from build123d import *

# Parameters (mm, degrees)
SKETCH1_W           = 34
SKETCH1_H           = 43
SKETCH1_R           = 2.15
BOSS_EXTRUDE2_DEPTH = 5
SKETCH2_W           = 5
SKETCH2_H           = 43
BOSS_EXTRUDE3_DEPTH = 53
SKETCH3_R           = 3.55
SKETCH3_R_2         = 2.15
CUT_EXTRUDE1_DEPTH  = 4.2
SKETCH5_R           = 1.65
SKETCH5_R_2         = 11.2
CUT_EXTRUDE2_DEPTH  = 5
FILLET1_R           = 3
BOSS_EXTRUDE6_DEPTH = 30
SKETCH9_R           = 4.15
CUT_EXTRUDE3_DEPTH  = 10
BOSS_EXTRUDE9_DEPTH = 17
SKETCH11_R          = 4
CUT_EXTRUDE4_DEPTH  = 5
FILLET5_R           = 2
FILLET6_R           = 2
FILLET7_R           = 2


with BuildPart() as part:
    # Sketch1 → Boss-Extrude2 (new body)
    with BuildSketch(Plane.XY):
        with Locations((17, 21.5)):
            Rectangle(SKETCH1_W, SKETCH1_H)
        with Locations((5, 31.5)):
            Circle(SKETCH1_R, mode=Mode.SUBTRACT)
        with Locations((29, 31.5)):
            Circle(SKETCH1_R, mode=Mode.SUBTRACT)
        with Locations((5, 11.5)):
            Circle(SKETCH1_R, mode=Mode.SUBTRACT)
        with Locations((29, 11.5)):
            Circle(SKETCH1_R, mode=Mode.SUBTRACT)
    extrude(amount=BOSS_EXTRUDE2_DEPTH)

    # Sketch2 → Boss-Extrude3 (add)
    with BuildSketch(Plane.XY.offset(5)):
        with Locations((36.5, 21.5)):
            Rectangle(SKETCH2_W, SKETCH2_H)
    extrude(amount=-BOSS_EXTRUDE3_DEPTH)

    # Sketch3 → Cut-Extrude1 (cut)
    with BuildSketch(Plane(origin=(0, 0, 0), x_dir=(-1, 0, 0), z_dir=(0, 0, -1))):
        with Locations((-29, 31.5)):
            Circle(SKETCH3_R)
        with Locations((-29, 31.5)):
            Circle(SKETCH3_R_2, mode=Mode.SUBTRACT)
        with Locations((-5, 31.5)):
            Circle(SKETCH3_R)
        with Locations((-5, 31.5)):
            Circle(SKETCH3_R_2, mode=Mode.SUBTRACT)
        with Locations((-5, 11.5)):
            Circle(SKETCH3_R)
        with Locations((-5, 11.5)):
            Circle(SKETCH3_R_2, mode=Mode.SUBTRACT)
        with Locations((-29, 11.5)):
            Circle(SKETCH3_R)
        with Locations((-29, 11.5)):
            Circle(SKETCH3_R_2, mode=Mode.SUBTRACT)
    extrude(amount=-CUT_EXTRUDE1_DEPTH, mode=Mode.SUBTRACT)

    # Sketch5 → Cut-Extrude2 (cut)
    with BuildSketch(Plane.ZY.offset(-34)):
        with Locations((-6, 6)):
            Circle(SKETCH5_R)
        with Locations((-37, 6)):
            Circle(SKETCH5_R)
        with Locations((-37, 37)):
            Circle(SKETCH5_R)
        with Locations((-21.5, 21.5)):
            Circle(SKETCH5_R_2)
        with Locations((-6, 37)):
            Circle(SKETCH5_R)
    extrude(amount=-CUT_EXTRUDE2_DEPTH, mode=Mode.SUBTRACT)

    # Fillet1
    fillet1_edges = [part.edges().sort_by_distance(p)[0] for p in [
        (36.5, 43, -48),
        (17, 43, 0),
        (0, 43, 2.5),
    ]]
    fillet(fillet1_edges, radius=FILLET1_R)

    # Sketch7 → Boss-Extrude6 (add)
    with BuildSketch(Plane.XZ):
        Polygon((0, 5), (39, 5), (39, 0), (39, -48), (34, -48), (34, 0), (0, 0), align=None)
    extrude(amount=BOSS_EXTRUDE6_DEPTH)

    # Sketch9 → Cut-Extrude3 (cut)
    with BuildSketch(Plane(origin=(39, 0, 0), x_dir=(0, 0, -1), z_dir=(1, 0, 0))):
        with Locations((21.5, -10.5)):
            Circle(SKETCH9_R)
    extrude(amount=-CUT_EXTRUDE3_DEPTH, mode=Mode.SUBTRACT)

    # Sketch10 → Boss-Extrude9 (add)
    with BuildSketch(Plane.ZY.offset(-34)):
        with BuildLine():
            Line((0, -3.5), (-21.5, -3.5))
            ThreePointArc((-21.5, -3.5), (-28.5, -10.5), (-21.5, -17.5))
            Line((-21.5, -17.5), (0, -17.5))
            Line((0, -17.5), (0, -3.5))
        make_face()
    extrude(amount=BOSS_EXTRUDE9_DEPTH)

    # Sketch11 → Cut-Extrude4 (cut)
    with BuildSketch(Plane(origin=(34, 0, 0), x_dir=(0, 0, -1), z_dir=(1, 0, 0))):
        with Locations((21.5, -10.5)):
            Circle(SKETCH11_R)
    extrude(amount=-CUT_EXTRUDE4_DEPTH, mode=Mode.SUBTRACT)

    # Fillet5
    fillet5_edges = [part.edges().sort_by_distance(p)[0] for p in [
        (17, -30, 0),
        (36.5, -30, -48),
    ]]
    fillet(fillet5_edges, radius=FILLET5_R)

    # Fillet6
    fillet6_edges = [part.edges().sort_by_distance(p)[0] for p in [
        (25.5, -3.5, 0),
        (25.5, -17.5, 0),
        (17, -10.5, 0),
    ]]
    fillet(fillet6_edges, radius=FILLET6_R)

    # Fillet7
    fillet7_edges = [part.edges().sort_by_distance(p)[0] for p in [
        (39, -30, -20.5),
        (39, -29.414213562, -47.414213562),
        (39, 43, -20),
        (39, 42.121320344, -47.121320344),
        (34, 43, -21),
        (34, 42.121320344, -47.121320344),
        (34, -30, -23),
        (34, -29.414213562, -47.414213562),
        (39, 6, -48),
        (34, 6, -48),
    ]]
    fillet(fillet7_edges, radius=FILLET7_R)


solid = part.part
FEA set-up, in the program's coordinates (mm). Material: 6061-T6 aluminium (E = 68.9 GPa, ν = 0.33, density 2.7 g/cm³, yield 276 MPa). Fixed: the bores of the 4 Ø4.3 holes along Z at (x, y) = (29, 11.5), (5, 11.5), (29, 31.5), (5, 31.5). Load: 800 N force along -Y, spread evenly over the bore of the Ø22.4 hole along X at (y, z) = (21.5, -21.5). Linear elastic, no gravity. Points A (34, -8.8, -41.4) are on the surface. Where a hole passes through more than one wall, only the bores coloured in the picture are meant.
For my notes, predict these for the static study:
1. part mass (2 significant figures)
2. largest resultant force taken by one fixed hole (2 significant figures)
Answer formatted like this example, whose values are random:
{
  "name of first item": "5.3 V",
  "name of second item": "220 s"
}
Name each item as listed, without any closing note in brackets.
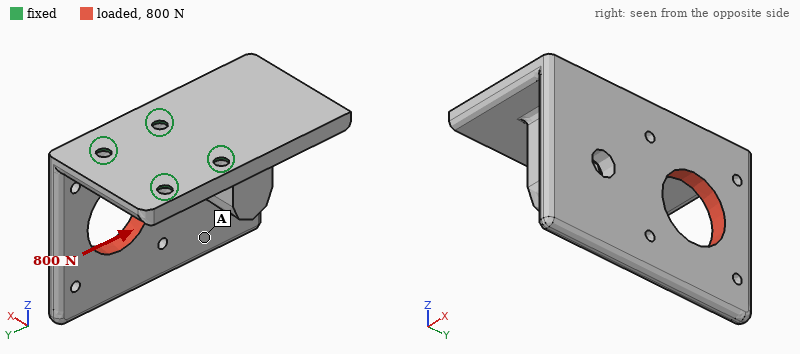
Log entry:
{
  "part mass": "93 g",
  "largest resultant force taken by one fixed hole": "1.0 kN"
}
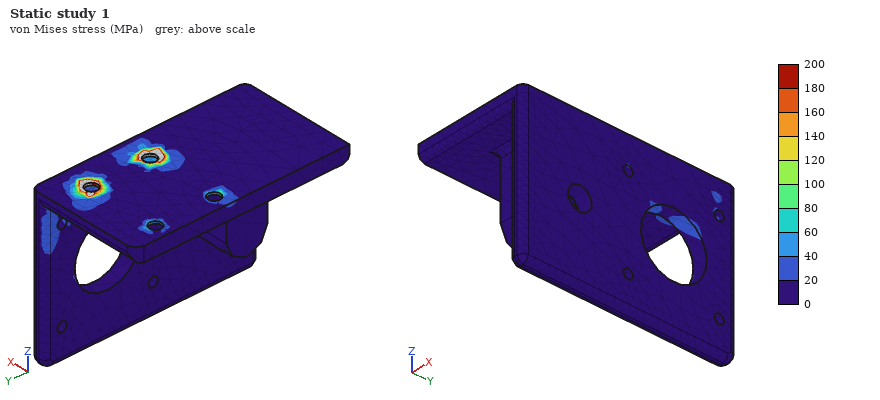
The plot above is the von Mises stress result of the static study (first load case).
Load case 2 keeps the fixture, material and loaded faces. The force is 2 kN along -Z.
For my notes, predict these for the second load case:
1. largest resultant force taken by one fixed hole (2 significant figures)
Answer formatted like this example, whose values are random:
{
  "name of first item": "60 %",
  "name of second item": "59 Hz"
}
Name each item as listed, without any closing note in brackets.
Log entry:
{
  "largest resultant force taken by one fixed hole": "1.4 kN"
}
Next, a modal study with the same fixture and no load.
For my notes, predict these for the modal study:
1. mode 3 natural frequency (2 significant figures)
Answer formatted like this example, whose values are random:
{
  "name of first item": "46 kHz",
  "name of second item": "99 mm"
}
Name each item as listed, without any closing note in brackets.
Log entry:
{
  "mode 3 natural frequency": "2900 Hz"
}
